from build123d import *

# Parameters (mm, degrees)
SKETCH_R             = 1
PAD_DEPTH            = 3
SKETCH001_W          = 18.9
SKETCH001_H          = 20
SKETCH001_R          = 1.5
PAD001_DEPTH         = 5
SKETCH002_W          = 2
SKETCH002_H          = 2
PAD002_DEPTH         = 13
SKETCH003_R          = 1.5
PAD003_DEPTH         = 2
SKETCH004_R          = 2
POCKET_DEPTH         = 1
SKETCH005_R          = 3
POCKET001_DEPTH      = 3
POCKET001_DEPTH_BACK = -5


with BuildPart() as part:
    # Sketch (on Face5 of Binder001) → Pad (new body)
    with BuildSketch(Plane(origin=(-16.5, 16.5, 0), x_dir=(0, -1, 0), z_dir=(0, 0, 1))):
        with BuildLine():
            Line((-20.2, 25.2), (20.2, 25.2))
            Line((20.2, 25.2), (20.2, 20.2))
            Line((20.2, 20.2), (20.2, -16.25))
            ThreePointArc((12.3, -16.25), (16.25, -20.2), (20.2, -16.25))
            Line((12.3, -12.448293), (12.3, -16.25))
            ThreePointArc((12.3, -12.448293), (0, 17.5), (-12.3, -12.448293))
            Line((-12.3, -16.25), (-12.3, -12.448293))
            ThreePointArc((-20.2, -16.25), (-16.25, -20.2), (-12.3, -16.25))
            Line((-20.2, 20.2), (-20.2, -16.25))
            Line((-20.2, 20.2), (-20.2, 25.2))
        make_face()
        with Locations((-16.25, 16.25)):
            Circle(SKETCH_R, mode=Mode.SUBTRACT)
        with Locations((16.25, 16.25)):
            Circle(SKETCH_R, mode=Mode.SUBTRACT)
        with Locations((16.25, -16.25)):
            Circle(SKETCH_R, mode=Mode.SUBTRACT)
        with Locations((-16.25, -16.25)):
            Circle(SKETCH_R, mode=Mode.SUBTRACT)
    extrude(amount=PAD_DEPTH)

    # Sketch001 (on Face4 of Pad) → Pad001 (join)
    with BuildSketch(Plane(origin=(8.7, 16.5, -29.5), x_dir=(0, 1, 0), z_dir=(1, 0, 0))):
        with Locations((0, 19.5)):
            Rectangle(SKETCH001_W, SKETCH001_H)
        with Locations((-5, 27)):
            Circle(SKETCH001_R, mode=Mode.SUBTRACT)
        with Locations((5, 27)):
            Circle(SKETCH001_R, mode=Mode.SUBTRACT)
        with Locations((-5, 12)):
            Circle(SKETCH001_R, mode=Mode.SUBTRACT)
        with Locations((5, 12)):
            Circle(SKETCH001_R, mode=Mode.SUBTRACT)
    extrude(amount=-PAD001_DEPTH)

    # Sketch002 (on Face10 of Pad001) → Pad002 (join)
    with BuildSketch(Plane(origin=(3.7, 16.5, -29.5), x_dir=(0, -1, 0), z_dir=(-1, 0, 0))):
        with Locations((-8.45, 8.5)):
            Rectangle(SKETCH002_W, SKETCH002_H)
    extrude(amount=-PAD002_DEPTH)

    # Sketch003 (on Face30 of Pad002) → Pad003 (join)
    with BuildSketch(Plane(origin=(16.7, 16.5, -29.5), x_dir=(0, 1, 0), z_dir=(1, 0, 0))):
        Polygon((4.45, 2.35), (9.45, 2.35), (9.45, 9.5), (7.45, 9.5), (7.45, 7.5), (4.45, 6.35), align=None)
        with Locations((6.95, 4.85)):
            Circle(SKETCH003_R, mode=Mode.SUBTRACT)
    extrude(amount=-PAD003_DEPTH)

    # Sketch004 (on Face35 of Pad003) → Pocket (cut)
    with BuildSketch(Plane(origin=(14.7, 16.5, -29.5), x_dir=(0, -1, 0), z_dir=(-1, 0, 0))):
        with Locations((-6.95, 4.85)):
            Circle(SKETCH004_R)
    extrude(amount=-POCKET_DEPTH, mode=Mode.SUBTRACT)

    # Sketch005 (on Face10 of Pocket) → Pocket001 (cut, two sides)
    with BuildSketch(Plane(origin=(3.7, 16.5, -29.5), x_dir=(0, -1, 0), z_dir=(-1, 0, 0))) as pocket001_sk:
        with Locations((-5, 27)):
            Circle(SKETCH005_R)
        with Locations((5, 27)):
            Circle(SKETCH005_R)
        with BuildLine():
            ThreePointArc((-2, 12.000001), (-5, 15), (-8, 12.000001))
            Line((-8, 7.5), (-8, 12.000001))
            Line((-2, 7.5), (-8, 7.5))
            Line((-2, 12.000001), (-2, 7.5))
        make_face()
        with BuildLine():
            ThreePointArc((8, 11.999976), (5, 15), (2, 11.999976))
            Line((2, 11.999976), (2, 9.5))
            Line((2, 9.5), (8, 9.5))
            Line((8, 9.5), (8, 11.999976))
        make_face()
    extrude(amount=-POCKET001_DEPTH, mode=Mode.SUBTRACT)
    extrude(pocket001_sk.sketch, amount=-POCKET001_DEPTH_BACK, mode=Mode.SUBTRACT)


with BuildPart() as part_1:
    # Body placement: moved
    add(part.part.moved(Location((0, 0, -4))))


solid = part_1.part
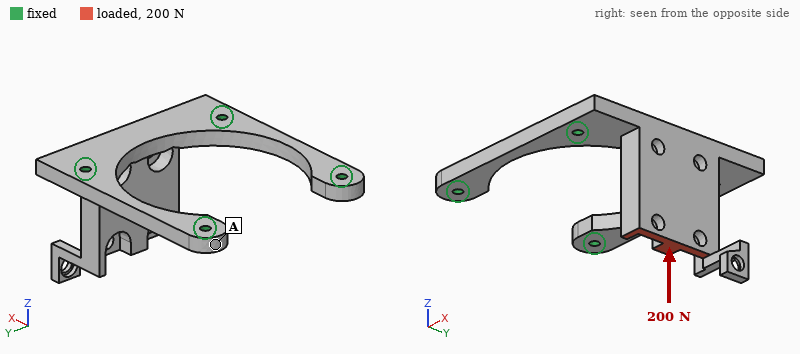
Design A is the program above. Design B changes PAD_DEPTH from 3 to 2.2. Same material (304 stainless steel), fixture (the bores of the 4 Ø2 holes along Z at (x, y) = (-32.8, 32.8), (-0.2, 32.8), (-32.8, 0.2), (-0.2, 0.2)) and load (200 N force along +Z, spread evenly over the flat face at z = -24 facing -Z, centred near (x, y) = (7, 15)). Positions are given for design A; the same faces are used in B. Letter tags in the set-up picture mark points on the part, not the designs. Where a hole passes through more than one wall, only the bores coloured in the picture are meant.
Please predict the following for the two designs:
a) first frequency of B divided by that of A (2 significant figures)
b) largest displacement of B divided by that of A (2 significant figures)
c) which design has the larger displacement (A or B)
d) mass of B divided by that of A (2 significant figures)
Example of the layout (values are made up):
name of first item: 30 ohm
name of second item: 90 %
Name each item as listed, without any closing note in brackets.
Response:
first frequency of B divided by that of A: 0.72
largest displacement of B divided by that of A: 2.1
which design has the larger displacement: B
mass of B divided by that of A: 0.84
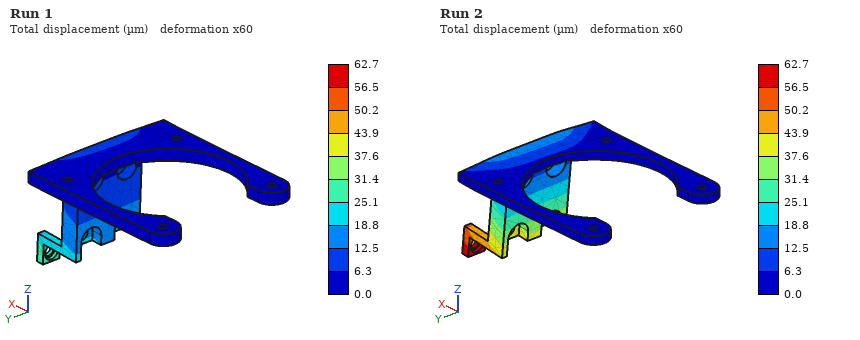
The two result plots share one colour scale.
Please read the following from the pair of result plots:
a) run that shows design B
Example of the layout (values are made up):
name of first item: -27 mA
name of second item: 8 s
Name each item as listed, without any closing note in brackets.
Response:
run that shows design B: Run 2
